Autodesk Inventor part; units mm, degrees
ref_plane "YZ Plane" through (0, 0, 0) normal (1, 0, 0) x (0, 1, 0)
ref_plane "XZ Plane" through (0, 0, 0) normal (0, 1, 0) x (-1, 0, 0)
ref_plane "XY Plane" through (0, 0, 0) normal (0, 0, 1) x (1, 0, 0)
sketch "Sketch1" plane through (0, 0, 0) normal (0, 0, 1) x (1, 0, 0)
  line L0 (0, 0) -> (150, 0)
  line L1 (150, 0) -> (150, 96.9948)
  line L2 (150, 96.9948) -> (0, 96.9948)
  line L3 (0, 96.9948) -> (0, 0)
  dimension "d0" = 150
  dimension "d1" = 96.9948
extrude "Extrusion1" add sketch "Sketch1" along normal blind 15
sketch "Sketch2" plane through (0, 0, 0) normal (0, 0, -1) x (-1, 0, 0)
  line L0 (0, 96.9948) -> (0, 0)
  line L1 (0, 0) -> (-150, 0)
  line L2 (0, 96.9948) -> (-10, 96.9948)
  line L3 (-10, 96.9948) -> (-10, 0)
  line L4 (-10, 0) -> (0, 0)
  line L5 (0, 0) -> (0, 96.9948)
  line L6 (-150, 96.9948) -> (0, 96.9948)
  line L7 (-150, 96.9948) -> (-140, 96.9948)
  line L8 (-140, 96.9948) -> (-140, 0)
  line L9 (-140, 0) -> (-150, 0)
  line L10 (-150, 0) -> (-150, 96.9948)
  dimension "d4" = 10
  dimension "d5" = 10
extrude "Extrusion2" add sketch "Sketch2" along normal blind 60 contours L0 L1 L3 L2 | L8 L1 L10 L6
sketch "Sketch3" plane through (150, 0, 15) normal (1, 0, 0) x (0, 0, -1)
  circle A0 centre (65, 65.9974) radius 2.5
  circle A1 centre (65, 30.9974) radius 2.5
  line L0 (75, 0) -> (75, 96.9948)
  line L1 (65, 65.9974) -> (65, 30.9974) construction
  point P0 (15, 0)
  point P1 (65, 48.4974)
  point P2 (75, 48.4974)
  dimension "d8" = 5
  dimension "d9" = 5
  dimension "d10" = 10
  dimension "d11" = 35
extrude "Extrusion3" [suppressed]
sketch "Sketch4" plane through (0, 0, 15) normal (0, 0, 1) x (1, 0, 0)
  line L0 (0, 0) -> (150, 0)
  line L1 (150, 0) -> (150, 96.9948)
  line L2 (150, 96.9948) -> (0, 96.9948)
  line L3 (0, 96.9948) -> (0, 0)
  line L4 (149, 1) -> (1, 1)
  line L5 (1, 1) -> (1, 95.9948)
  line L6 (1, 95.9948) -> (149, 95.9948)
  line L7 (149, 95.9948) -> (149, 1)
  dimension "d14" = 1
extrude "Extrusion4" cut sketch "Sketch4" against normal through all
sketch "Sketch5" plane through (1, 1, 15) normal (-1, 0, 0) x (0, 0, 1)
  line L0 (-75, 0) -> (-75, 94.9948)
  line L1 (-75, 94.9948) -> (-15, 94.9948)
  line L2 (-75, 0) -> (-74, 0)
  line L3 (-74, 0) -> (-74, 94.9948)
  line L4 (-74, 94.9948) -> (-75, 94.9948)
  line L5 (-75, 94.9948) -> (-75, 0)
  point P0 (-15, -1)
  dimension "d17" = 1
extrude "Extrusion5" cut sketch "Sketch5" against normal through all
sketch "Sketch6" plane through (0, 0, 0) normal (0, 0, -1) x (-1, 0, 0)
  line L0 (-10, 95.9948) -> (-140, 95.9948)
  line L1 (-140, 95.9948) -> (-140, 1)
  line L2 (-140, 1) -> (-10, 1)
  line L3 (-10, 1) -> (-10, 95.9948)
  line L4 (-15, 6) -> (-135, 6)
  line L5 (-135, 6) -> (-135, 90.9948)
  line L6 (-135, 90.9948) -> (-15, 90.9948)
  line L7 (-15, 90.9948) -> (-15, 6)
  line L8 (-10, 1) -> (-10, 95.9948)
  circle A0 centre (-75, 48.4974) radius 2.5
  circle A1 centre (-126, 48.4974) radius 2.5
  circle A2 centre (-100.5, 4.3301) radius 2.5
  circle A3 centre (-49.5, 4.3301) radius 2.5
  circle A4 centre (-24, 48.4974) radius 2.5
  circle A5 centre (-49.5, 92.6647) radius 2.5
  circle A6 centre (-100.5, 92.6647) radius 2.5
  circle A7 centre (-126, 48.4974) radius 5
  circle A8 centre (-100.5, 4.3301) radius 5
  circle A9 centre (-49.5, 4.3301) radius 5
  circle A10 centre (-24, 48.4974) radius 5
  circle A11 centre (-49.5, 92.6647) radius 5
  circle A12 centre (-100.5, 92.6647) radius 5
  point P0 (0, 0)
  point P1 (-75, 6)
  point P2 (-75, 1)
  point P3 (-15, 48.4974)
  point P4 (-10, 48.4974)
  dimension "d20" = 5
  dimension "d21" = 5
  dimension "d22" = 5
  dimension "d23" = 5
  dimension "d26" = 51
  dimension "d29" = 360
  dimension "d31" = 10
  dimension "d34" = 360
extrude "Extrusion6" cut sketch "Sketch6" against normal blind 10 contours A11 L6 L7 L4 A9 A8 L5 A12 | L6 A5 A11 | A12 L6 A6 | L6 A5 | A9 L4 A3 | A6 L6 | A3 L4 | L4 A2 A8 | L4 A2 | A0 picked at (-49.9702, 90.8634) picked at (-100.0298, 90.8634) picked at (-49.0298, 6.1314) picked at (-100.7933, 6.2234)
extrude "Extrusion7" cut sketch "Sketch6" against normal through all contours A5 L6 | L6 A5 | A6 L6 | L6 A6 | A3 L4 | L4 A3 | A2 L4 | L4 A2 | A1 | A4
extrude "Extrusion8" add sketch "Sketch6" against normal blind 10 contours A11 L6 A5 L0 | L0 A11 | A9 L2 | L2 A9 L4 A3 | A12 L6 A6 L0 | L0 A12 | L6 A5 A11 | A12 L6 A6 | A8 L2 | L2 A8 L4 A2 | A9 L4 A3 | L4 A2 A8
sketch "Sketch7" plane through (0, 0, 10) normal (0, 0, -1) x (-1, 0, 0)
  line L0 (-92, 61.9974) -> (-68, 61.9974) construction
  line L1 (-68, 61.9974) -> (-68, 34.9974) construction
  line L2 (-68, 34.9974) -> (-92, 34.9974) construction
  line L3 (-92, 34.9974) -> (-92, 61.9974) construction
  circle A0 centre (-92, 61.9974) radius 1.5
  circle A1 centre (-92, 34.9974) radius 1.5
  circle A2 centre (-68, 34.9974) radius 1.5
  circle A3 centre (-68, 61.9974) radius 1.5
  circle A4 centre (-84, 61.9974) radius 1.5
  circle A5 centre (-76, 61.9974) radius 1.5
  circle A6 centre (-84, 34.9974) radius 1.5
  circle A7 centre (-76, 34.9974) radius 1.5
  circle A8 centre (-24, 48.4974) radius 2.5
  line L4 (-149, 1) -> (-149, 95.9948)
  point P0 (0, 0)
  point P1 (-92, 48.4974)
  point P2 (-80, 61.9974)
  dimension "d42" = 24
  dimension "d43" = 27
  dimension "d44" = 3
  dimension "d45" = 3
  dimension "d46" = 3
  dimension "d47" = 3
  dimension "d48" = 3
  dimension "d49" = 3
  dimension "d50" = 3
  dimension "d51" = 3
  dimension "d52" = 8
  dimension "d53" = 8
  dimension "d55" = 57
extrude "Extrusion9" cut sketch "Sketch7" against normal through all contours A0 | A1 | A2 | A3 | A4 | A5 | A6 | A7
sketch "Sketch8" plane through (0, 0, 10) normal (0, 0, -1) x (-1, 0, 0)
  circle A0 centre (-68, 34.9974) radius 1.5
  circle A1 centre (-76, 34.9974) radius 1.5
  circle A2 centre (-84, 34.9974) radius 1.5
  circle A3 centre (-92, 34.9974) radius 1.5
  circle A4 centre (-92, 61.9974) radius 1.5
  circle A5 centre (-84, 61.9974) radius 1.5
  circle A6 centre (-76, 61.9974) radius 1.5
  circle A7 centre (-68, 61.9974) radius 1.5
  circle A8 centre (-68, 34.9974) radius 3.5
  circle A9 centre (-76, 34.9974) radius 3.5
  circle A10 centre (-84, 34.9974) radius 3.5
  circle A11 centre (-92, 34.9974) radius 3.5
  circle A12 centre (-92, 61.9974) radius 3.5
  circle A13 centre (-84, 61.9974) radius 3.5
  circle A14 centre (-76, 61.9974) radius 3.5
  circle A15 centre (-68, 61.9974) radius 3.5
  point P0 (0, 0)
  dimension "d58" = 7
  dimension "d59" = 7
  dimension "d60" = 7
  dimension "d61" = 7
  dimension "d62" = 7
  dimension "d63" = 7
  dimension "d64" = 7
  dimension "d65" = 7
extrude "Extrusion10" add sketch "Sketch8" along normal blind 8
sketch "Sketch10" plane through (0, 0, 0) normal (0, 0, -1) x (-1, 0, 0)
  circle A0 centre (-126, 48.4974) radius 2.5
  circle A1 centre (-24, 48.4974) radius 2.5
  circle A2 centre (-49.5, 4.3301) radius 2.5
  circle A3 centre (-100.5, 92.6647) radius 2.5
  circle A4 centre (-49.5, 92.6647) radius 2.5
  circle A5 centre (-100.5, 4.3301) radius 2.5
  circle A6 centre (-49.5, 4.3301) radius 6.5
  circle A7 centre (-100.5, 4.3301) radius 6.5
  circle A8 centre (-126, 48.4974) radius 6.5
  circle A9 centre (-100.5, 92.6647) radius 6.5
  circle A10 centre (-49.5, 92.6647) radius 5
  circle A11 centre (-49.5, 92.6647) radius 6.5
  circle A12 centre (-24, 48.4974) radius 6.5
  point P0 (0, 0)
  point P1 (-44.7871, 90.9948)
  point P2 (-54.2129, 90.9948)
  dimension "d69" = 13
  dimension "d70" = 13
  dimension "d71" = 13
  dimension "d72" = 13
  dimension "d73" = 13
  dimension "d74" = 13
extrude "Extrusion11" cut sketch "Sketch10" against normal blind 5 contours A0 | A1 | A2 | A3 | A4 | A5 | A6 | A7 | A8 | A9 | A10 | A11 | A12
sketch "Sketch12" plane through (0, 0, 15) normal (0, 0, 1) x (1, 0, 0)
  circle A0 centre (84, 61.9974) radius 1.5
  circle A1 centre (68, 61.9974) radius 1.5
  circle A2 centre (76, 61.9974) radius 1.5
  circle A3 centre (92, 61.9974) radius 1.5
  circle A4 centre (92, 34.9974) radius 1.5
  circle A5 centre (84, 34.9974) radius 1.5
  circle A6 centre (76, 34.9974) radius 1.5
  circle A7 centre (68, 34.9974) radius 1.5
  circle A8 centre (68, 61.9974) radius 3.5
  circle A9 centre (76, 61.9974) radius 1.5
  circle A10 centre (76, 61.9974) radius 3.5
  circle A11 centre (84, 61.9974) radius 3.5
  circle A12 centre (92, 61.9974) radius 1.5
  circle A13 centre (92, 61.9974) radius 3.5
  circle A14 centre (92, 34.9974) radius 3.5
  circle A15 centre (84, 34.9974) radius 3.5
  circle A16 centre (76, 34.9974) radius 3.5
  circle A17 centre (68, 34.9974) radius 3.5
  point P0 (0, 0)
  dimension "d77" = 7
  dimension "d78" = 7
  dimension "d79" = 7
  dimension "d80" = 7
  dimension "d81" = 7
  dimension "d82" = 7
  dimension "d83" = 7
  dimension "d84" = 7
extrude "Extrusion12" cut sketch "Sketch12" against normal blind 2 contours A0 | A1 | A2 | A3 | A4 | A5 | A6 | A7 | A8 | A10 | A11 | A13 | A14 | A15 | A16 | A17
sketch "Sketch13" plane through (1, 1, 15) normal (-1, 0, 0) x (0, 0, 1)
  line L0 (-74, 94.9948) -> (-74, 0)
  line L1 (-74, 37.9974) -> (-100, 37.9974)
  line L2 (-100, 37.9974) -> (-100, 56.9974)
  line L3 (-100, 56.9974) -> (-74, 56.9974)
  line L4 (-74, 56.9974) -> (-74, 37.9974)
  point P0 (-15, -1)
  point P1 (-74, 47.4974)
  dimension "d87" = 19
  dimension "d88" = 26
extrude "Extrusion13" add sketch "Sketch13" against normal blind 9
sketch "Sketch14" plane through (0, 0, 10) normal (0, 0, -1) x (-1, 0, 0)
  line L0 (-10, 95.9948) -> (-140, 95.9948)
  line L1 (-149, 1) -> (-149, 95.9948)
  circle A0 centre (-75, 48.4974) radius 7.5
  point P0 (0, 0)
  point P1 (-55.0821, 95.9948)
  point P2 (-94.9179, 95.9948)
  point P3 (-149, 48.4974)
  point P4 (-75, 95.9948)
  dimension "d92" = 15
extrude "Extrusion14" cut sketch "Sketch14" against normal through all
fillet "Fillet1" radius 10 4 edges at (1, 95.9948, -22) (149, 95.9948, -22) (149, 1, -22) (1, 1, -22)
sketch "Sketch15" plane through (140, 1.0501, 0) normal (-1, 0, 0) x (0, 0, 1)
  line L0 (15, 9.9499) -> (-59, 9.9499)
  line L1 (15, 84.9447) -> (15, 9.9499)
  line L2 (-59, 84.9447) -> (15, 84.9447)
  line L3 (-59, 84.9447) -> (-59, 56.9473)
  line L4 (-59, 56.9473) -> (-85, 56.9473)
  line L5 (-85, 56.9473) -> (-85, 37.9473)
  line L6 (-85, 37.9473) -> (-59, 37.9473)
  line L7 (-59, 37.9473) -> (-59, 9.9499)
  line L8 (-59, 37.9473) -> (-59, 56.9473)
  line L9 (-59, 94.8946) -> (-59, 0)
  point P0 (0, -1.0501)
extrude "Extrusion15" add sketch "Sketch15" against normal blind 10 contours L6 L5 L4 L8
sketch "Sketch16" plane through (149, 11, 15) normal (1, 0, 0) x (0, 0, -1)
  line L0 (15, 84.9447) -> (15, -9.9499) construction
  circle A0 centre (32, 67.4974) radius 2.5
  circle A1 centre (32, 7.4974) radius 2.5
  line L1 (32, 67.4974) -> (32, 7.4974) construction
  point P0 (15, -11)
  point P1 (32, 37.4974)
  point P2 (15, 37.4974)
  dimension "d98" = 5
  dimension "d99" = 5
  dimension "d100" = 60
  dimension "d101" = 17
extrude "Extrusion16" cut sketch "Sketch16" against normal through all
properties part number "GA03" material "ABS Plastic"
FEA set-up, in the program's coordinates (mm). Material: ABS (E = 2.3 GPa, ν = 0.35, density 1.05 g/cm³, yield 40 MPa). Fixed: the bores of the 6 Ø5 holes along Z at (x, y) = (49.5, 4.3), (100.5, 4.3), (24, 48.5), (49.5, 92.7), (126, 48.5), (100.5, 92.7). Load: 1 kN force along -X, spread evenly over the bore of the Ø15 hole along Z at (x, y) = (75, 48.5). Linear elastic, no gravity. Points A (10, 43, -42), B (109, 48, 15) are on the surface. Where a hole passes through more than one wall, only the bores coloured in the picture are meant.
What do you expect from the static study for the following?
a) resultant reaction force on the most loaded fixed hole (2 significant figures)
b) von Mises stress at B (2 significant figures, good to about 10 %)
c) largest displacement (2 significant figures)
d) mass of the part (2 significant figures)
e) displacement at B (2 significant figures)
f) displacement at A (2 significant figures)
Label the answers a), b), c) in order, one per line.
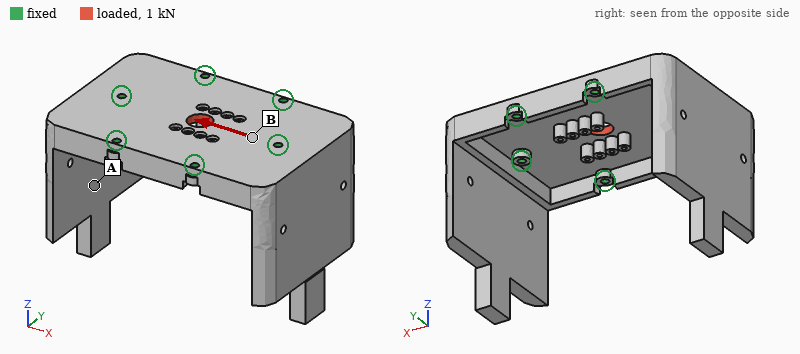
a) 250 N
b) 2.3 MPa
c) 57 µm
d) 220 g
e) 16 µm
f) 23 µm
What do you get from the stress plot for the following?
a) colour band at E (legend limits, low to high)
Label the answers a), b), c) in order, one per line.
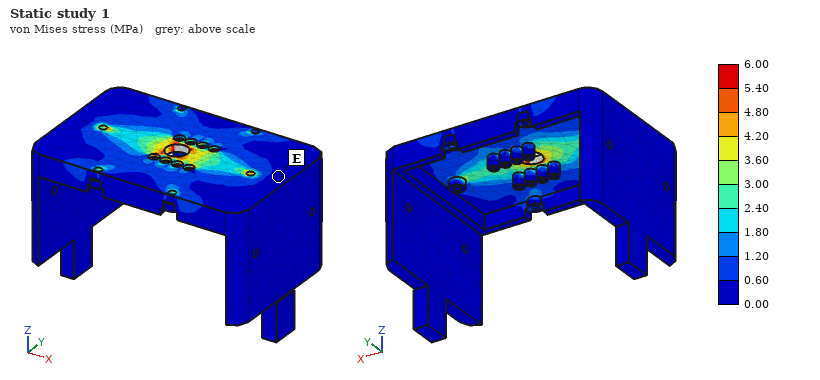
a) 0.00 to 0.60 MPa
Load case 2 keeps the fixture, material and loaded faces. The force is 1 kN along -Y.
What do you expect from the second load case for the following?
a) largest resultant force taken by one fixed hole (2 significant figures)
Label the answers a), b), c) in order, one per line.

a) 230 N
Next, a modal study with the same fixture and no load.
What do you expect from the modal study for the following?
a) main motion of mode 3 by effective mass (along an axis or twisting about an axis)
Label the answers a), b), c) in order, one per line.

a) along Y
